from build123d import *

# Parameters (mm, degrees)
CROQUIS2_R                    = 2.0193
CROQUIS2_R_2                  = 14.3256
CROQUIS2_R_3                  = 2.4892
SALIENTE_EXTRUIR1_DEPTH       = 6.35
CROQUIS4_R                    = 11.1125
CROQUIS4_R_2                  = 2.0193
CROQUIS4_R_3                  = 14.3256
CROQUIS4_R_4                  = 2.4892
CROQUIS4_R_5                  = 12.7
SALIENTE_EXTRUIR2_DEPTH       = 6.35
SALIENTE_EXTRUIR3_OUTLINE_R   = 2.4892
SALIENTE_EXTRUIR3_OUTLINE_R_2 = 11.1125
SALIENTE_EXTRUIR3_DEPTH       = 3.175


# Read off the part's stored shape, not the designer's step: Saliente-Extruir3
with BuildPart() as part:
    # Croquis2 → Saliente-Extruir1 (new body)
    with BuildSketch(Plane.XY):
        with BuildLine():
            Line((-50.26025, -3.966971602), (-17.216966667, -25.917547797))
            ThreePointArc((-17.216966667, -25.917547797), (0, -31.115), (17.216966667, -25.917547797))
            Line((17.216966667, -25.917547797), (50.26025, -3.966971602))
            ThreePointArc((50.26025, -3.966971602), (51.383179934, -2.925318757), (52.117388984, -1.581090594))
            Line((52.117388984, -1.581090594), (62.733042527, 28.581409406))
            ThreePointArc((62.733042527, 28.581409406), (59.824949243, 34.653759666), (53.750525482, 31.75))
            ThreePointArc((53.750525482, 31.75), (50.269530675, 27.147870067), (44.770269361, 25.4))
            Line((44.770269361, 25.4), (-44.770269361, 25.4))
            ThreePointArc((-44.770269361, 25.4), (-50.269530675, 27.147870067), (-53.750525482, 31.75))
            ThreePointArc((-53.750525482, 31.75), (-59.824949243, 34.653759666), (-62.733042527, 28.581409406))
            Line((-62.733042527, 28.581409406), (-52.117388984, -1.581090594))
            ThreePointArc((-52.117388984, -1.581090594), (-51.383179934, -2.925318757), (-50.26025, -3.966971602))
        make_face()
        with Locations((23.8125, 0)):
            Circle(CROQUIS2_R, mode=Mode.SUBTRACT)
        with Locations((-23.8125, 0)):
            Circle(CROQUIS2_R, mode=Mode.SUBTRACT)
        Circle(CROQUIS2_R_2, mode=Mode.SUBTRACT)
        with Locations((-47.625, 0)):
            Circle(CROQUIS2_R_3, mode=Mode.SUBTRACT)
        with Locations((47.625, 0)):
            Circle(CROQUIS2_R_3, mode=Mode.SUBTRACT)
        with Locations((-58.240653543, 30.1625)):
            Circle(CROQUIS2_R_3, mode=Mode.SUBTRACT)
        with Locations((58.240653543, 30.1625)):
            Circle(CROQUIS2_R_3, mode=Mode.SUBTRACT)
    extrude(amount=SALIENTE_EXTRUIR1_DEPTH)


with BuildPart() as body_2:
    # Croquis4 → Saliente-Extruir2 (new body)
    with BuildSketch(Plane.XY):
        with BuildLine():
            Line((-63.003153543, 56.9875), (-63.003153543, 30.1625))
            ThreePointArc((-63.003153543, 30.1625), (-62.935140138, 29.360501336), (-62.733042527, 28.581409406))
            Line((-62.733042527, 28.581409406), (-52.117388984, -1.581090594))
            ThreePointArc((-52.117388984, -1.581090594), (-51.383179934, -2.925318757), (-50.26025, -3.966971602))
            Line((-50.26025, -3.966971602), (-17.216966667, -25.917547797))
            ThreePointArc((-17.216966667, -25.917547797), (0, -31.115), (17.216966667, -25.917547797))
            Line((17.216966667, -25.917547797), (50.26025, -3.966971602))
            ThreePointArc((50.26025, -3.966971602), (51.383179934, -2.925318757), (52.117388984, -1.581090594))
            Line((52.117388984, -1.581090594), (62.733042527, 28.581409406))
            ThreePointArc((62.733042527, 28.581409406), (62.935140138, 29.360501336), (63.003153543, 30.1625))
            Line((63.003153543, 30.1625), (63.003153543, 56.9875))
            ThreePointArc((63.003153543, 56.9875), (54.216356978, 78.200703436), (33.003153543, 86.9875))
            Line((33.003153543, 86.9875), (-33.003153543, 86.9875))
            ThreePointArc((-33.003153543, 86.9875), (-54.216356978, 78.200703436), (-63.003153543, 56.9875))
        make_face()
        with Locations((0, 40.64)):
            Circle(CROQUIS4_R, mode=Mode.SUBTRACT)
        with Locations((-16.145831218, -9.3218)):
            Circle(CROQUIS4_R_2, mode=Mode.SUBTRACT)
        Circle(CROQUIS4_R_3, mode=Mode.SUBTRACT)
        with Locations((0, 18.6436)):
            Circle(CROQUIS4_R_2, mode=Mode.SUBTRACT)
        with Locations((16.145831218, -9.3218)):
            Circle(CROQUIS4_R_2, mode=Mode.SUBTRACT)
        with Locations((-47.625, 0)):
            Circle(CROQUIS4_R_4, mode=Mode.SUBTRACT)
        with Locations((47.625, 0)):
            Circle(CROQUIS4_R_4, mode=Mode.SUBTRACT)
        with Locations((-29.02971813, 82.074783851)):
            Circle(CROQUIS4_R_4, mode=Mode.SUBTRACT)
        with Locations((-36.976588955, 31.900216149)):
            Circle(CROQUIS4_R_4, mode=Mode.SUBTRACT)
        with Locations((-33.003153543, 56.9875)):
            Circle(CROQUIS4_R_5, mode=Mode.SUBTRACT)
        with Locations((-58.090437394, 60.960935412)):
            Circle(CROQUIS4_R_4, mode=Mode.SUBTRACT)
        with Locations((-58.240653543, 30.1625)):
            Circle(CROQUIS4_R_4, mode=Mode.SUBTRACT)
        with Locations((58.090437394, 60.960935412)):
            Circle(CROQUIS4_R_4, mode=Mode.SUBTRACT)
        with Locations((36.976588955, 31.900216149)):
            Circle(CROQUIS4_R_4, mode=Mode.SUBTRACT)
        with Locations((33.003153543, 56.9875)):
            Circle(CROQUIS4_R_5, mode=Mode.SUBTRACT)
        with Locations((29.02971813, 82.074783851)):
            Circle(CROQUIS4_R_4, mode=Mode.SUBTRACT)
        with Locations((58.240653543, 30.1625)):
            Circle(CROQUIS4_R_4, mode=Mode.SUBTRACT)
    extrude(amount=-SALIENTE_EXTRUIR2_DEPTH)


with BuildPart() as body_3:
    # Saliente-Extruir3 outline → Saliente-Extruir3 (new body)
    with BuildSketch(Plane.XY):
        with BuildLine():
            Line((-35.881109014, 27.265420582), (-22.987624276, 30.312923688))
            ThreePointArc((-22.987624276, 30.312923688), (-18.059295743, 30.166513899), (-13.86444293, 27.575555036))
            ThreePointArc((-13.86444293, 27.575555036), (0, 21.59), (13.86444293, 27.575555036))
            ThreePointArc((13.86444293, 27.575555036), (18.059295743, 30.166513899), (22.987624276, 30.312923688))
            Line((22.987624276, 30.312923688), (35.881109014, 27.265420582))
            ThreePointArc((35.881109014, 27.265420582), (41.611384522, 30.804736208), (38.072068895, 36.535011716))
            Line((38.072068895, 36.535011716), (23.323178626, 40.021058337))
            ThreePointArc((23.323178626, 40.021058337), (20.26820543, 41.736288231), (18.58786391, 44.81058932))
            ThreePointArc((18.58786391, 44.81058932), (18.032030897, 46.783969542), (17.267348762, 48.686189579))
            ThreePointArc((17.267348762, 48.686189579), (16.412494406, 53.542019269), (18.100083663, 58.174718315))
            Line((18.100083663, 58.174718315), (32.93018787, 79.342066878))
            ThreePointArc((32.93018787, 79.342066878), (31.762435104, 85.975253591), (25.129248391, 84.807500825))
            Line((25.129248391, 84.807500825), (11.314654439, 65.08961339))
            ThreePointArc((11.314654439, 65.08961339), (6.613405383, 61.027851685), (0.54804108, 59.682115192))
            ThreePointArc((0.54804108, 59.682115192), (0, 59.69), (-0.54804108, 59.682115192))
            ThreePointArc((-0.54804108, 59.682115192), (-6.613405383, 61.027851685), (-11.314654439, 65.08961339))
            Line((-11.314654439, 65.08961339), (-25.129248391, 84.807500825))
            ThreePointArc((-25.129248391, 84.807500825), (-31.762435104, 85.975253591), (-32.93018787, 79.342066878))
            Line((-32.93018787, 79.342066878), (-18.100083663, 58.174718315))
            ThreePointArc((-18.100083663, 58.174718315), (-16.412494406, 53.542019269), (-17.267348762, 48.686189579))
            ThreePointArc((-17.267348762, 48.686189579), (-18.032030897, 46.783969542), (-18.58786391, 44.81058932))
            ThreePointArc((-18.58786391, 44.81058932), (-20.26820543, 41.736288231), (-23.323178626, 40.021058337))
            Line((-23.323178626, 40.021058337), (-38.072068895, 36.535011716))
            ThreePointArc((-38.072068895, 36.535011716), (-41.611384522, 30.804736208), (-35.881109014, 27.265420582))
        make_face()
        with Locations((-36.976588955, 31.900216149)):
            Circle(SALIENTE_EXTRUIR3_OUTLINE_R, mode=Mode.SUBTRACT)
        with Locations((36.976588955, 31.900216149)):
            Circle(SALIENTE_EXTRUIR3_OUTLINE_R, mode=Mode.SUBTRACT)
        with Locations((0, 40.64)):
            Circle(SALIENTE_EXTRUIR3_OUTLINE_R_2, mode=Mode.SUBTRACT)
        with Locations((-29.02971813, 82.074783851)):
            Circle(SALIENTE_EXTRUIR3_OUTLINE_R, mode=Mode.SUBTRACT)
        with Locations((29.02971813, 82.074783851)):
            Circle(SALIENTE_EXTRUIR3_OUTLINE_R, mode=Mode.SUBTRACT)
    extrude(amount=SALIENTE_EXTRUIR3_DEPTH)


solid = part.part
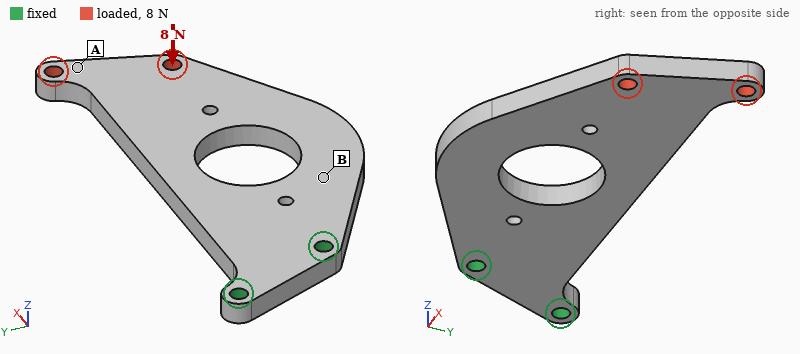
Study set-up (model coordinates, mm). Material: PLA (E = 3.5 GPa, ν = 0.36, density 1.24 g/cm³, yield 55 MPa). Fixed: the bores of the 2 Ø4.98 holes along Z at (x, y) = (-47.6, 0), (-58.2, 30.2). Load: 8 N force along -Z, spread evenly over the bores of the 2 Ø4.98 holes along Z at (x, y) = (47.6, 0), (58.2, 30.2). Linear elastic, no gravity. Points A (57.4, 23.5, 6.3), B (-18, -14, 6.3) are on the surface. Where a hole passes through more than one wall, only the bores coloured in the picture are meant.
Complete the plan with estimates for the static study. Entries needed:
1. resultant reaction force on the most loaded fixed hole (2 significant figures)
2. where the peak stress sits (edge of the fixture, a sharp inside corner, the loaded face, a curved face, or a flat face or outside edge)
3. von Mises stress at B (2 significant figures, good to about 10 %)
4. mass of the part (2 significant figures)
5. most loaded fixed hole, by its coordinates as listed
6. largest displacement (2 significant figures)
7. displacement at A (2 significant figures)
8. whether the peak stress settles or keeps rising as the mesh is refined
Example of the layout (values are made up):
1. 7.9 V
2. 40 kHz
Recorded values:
1. 15 N
2. edge of the fixture
3. 2.1 MPa
4. 34 g
5. (-47.6, 0)
6. 1.4 mm
7. 1.3 mm
8. keeps rising
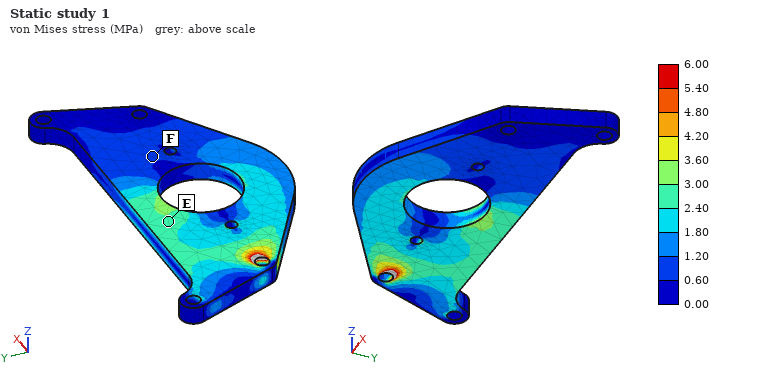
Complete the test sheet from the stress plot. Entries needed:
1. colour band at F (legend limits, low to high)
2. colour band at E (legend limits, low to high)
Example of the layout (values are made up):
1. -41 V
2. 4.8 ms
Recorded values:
1. 0.60 to 1.20 MPa
2. 2.40 to 3.00 MPa
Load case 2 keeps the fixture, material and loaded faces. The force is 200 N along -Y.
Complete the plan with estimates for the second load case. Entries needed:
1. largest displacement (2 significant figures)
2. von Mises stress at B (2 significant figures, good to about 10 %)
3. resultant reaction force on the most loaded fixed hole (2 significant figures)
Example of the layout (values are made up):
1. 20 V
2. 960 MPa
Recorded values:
1. 1.4 mm
2. 4.4 MPa
3. 730 N
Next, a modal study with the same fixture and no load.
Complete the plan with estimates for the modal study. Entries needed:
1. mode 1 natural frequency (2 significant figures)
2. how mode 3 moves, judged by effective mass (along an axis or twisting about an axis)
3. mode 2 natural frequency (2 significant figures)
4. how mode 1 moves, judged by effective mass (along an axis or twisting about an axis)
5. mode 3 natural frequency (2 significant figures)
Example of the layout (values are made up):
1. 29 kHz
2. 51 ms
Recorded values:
1. 140 Hz
2. along Y
3. 510 Hz
4. along Z
5. 620 Hz
